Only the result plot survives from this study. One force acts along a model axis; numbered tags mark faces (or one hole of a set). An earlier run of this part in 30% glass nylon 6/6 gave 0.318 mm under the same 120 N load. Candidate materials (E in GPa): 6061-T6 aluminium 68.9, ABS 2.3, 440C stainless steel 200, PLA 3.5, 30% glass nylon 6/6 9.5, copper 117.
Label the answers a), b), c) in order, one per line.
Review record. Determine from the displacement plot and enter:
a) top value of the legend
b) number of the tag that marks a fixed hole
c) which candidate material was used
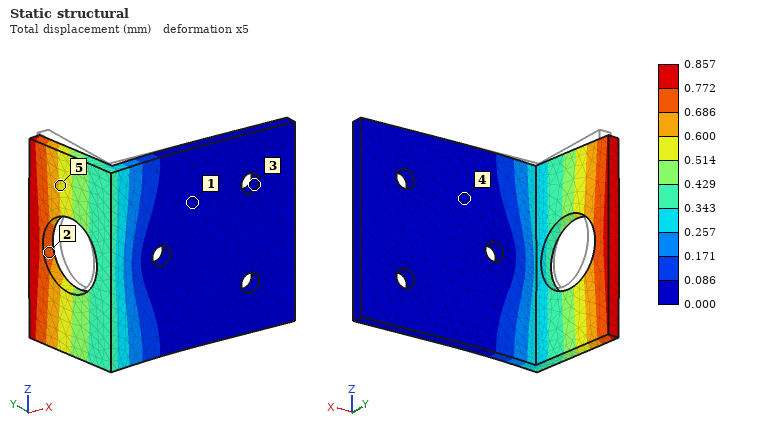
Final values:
a) 0.857 mm
b) 3
c) PLA
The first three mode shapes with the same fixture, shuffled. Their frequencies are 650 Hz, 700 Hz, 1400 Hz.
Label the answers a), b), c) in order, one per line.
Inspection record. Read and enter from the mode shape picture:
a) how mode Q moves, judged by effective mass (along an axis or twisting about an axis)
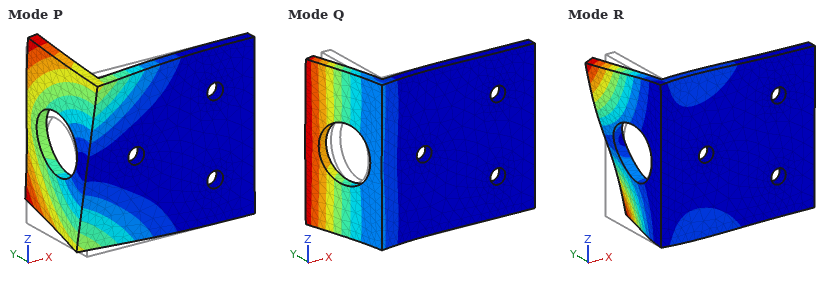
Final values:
a) along X
